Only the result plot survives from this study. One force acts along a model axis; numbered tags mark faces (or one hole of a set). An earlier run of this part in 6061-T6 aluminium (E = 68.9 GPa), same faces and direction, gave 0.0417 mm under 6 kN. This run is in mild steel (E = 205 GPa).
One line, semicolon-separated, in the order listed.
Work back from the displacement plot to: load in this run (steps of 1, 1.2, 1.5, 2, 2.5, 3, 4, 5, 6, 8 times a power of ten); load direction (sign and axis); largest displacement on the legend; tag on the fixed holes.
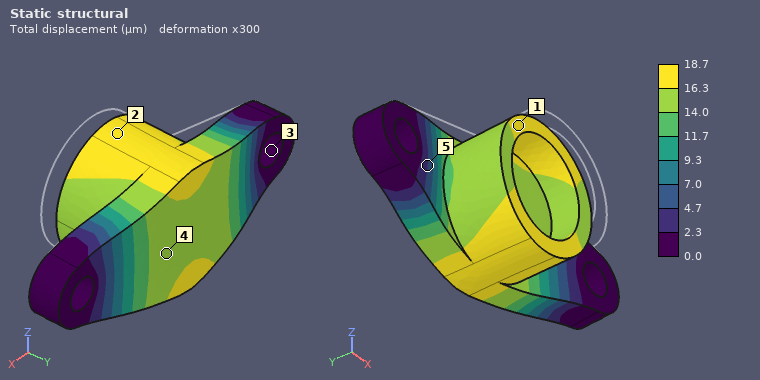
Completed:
8 kN; +Y; 18.7 µm; 3
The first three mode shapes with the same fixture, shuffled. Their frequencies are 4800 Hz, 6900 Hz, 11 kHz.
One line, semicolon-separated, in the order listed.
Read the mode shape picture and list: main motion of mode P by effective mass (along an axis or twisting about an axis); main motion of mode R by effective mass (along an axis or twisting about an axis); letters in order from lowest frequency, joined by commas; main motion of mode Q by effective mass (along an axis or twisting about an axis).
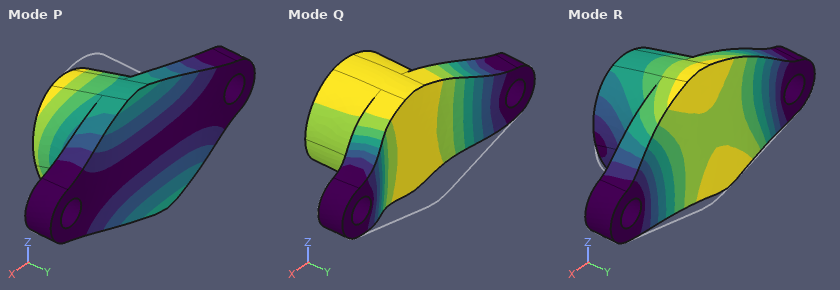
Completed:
along Z; along Z; P, Q, R; along Y
